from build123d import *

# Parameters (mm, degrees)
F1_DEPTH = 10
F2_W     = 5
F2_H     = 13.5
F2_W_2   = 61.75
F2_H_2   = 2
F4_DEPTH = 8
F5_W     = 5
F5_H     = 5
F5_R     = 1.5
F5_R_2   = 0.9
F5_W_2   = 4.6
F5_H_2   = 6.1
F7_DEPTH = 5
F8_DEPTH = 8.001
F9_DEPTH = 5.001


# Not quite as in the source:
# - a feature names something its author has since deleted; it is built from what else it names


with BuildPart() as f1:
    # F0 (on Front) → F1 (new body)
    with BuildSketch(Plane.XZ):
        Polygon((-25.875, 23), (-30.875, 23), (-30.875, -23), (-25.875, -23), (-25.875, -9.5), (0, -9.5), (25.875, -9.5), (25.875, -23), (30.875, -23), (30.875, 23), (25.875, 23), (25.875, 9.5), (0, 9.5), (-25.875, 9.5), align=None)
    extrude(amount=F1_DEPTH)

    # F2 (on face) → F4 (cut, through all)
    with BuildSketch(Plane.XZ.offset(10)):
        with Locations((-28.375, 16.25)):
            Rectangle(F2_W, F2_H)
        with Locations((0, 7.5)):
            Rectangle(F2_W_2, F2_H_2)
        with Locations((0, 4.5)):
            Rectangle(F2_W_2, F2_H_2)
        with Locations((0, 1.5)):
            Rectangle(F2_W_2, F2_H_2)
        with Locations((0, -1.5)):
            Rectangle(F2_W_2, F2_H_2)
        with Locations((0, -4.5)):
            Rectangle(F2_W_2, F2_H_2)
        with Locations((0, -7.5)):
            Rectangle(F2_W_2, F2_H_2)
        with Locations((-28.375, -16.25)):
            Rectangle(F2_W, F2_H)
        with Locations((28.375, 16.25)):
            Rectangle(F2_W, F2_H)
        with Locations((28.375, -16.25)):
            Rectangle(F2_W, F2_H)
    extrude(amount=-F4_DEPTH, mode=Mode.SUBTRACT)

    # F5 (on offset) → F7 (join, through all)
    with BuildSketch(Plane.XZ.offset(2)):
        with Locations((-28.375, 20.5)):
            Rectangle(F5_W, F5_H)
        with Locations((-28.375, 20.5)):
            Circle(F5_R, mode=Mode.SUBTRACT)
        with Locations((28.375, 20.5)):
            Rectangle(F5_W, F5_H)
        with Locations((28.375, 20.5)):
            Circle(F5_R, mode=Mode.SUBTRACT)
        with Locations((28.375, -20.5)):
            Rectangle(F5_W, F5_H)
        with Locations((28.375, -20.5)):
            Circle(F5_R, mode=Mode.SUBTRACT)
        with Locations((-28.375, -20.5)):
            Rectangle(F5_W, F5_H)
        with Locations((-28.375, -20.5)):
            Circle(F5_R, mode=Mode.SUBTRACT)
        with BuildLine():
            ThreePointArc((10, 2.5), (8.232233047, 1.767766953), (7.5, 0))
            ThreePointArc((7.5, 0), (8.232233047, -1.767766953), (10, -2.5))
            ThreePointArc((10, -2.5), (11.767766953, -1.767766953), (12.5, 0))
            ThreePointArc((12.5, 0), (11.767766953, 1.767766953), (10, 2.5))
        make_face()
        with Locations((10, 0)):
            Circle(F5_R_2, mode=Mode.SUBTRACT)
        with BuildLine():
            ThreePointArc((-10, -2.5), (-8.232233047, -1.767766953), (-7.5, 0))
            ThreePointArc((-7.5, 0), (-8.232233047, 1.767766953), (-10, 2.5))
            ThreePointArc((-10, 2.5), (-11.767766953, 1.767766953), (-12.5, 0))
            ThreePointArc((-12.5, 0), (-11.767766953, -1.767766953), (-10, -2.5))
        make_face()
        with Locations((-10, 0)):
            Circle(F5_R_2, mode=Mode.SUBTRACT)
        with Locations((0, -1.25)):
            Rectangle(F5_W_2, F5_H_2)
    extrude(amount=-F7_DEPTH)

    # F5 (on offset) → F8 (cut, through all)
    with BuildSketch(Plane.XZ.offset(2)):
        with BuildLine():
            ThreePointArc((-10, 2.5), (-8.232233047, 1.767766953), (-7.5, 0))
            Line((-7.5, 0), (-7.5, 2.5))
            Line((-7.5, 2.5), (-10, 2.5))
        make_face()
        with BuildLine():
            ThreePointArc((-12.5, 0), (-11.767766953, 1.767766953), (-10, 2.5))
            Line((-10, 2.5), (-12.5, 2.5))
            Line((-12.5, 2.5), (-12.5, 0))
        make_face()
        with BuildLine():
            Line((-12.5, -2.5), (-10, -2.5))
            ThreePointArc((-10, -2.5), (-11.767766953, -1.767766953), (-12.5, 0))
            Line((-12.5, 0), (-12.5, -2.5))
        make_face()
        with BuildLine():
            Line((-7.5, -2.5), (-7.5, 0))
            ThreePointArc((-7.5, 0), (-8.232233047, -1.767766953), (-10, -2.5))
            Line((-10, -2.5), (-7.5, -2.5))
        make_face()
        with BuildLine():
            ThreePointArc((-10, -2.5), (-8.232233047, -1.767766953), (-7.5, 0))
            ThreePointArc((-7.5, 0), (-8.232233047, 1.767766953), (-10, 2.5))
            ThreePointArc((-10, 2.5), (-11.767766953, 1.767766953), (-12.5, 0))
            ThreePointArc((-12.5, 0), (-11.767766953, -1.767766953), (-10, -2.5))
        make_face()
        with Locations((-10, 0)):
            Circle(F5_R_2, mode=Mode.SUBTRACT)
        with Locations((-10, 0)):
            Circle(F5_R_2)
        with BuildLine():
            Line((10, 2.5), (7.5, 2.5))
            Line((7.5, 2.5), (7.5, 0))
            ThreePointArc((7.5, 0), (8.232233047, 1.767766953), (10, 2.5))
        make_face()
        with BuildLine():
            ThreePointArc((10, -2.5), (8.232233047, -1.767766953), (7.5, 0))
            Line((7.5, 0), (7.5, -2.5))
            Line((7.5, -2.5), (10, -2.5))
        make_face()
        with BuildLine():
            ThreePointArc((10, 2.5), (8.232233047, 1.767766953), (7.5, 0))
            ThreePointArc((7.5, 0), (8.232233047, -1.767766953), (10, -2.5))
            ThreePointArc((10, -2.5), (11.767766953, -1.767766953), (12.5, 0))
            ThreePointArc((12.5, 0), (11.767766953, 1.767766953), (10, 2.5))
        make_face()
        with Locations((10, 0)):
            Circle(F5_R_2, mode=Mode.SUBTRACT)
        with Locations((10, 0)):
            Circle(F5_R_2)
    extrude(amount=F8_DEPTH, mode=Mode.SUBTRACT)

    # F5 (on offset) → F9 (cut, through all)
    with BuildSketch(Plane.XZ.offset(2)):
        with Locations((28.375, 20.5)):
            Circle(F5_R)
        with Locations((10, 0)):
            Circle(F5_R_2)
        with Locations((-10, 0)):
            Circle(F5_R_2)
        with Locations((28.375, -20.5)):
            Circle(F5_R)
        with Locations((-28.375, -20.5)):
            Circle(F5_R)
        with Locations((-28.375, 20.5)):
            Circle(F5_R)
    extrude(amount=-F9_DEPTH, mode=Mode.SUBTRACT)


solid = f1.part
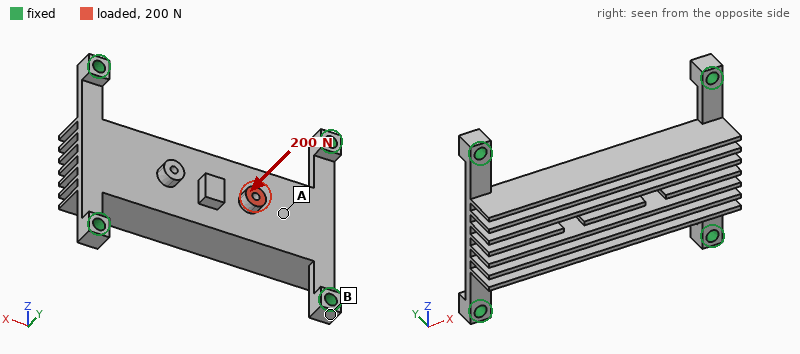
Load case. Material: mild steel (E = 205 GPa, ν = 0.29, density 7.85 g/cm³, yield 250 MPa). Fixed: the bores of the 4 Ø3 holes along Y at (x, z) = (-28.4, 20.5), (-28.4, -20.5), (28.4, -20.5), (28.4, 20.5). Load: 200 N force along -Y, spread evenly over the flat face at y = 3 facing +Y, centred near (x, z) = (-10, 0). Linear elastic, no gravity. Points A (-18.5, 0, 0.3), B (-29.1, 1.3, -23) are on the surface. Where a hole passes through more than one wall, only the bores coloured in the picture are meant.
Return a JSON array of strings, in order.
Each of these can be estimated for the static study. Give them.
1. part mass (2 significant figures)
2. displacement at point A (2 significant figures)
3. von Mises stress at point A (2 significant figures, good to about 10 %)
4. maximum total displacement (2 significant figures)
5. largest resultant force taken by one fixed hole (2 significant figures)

["52 g", "24 µm", "28 MPa", "25 µm", "72 N"]
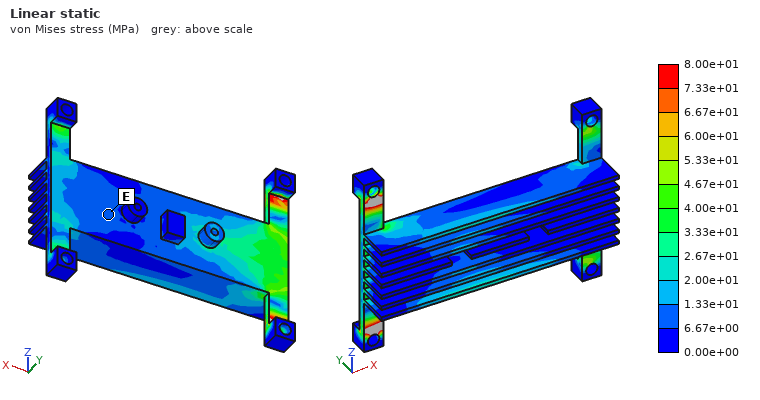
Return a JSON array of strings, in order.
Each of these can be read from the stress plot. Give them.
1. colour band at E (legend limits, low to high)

["6.67e+00 to 1.33e+01 MPa"]
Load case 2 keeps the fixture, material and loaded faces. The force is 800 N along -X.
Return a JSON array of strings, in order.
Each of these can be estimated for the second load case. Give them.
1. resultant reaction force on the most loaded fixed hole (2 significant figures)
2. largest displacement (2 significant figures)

["230 N", "26 µm"]
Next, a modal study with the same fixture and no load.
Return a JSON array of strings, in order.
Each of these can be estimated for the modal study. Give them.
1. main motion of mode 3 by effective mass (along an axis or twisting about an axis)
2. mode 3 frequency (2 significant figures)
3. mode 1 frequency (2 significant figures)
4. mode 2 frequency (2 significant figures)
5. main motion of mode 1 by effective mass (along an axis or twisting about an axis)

["along Z", "4600 Hz", "2600 Hz", "3900 Hz", "along Y"]
